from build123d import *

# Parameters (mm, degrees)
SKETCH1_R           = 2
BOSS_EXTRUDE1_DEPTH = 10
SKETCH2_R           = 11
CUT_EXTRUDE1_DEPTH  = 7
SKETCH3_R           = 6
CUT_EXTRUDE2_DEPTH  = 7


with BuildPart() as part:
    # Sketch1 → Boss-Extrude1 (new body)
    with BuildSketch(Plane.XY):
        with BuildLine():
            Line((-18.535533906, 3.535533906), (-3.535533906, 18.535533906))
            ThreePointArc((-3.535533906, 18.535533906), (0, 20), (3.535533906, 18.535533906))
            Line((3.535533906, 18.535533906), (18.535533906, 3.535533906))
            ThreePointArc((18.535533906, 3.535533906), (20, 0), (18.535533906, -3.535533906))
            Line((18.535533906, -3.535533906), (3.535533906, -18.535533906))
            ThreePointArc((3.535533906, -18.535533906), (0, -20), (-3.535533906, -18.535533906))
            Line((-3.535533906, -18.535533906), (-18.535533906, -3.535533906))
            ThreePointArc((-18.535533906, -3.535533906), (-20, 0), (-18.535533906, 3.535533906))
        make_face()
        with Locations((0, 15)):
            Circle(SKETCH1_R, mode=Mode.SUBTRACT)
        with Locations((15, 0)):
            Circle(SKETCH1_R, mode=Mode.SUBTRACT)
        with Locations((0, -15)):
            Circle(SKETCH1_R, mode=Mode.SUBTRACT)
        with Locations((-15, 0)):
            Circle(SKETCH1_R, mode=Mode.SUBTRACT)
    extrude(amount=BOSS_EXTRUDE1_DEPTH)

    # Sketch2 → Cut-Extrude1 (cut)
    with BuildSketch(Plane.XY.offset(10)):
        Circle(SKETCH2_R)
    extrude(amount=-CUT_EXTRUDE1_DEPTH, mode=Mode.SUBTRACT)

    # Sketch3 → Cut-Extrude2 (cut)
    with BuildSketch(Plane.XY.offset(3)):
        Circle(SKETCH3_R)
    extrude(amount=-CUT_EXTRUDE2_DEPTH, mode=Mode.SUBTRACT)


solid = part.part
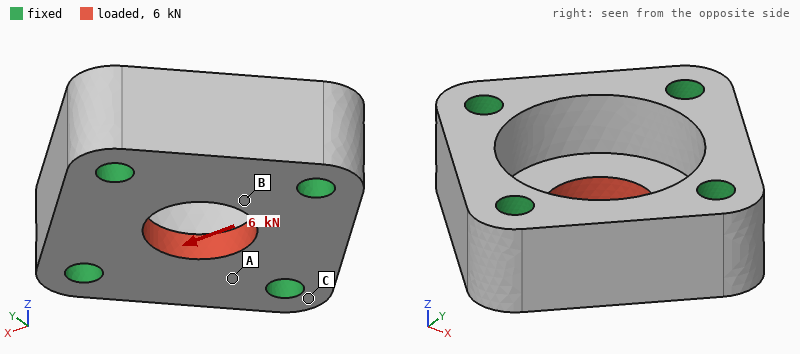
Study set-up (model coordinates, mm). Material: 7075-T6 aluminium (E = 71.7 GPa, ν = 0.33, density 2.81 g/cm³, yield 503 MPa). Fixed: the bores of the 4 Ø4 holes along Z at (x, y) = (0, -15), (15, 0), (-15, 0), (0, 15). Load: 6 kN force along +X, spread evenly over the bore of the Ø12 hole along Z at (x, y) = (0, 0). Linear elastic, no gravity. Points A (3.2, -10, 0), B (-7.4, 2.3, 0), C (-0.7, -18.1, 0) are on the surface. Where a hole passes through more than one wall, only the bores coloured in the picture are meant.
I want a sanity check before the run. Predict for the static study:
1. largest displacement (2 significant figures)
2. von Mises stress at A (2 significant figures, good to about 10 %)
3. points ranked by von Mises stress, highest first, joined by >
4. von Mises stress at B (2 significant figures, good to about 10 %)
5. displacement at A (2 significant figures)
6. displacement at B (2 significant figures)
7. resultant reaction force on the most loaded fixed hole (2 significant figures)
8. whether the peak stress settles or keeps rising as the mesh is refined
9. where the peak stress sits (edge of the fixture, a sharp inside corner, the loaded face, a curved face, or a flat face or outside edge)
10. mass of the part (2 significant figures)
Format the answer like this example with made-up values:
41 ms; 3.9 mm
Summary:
9.7 µm; 20 MPa; B > A > C; 65 MPa; 3.8 µm; 6.8 µm; 1.9 kN; keeps rising; edge of the fixture; 17 g
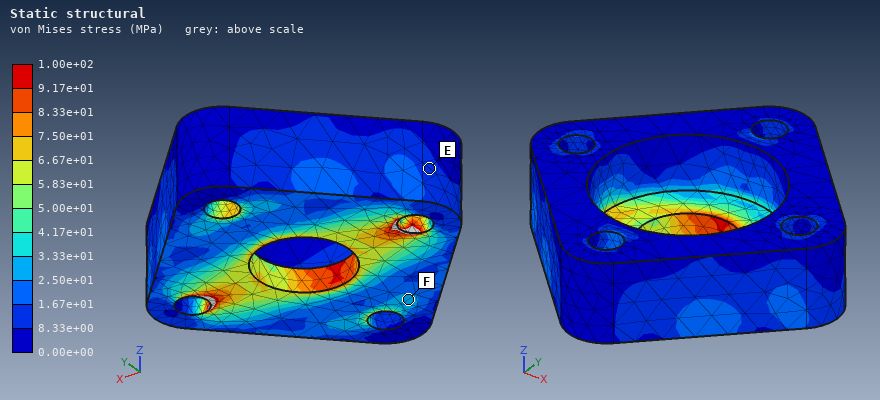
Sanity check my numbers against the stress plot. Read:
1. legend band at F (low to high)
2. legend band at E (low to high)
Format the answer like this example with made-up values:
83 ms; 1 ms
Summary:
2.50e+01 to 3.33e+01 MPa; 8.33e+00 to 1.67e+01 MPa
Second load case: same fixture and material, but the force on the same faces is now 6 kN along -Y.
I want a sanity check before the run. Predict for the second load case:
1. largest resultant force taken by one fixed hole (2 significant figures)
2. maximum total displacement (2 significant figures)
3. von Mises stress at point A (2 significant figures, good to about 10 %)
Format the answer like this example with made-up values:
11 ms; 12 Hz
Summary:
1.9 kN; 9.7 µm; 56 MPa
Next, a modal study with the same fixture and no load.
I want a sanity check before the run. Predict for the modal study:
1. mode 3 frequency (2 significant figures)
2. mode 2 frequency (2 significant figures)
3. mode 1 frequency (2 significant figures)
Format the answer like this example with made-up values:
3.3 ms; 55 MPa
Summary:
64 kHz; 59 kHz; 57 kHz
